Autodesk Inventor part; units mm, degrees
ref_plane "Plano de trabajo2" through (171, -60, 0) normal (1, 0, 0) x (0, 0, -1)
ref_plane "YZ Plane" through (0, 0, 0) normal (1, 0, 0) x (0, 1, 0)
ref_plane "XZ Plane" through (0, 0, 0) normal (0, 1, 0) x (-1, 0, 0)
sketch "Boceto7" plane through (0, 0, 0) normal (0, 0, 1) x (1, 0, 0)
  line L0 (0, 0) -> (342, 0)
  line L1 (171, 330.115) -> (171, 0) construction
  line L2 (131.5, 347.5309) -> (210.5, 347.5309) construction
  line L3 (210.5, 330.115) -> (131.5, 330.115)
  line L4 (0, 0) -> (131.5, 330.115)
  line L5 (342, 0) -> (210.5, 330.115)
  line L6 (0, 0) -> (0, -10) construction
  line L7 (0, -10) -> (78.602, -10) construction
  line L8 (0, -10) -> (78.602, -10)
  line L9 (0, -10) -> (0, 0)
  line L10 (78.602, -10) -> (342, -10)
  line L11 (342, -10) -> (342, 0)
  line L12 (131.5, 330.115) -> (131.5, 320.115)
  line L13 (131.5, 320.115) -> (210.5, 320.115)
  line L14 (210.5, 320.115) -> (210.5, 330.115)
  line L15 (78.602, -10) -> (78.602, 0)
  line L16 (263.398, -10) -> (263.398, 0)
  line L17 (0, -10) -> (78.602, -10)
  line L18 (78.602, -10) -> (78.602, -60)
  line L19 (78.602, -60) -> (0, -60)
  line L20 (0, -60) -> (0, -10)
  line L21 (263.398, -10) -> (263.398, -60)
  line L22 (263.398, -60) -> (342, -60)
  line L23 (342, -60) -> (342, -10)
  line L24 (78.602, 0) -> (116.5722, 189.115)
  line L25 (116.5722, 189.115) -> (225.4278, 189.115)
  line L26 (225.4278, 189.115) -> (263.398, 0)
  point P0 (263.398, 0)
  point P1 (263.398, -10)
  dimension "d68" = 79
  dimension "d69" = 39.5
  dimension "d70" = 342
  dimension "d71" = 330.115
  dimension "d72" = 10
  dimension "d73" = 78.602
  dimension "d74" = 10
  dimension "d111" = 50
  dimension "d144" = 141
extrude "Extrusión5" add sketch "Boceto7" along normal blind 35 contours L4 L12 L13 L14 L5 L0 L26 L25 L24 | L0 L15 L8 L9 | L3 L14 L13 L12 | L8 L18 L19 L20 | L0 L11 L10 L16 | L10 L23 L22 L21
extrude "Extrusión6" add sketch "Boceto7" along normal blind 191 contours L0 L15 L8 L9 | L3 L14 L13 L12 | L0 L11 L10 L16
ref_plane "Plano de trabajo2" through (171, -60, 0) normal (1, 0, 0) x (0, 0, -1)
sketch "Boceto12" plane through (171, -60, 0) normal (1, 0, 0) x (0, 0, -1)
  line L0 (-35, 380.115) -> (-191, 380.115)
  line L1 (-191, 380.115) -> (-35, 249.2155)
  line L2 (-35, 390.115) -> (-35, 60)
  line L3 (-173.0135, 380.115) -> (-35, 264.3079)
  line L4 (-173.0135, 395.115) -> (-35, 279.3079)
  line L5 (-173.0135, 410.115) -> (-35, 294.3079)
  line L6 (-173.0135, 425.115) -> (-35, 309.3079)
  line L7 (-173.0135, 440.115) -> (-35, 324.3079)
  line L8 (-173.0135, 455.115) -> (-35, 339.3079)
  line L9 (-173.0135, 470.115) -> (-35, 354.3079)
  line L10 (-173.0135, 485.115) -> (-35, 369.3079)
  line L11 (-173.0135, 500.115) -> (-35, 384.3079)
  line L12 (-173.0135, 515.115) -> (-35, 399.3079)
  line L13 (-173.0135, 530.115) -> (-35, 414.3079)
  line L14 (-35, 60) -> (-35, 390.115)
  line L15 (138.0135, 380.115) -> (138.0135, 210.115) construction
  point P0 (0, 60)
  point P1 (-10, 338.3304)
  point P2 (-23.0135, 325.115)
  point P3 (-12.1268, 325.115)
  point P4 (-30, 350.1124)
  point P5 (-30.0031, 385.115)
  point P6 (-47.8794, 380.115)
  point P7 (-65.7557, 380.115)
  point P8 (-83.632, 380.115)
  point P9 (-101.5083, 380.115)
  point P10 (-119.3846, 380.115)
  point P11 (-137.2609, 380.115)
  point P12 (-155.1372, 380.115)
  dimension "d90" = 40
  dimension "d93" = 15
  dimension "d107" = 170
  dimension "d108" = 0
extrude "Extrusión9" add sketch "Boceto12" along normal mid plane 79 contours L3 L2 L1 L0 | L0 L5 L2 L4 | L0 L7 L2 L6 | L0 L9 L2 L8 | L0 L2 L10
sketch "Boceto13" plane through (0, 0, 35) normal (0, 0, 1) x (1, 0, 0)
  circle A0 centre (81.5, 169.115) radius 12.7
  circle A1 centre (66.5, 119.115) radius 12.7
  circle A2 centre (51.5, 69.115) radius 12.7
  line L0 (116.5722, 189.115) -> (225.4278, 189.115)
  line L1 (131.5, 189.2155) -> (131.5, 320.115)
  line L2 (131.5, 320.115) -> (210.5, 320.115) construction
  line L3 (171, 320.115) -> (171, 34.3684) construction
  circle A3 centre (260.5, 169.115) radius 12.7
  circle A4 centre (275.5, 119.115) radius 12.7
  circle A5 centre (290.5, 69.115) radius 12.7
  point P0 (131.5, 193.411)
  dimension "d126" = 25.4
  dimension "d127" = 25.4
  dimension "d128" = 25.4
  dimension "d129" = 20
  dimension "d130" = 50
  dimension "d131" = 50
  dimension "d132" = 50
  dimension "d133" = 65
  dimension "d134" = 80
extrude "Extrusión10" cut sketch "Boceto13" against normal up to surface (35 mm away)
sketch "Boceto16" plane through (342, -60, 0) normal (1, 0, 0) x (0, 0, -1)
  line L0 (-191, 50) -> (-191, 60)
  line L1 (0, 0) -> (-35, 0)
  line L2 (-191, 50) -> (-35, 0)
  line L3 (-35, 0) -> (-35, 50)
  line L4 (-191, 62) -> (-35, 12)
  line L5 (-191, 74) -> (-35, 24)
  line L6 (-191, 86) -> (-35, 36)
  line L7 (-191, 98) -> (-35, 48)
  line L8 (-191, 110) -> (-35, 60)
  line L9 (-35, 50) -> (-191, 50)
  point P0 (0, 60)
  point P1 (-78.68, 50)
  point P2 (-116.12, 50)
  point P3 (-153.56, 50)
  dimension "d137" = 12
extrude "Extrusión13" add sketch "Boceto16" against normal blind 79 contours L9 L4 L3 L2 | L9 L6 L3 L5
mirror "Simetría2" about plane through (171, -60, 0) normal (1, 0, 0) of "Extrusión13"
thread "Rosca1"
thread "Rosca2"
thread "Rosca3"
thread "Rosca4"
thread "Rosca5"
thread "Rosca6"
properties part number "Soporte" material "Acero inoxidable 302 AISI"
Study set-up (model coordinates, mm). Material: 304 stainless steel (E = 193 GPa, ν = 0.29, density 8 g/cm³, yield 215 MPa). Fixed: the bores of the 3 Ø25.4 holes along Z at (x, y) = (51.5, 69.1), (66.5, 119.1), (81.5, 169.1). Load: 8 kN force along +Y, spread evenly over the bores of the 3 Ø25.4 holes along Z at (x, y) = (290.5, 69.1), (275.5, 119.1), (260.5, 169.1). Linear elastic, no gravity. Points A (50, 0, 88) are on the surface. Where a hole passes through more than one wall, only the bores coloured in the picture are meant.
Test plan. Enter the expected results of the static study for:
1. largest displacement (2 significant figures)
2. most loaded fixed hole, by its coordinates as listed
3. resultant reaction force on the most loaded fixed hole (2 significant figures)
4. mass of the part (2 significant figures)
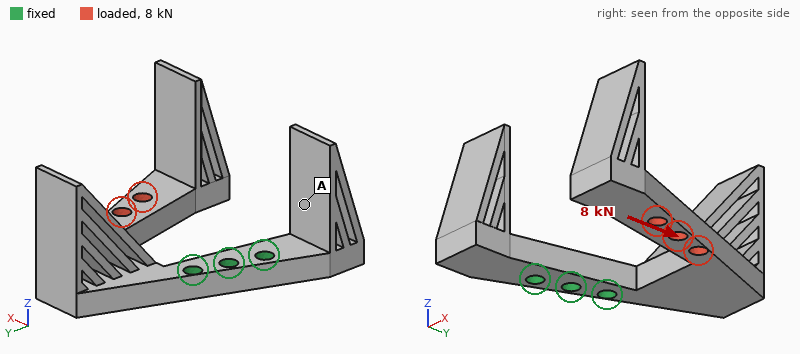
1.0 mm
(66.5, 119.1)
11 kN
23 kg
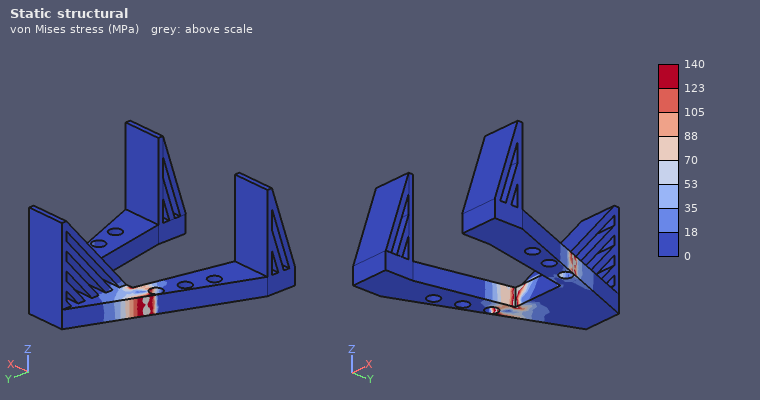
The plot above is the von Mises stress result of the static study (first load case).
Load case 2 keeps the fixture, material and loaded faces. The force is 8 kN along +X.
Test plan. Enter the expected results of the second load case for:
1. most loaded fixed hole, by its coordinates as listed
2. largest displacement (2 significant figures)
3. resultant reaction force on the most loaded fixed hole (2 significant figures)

(81.5, 169.1)
0.81 mm
5.8 kN
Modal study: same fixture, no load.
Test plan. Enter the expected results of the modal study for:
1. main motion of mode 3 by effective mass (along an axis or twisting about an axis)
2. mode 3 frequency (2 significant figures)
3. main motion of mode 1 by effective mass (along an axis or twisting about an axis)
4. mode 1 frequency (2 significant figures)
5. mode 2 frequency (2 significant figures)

along Z
250 Hz
along Z
95 Hz
120 Hz
